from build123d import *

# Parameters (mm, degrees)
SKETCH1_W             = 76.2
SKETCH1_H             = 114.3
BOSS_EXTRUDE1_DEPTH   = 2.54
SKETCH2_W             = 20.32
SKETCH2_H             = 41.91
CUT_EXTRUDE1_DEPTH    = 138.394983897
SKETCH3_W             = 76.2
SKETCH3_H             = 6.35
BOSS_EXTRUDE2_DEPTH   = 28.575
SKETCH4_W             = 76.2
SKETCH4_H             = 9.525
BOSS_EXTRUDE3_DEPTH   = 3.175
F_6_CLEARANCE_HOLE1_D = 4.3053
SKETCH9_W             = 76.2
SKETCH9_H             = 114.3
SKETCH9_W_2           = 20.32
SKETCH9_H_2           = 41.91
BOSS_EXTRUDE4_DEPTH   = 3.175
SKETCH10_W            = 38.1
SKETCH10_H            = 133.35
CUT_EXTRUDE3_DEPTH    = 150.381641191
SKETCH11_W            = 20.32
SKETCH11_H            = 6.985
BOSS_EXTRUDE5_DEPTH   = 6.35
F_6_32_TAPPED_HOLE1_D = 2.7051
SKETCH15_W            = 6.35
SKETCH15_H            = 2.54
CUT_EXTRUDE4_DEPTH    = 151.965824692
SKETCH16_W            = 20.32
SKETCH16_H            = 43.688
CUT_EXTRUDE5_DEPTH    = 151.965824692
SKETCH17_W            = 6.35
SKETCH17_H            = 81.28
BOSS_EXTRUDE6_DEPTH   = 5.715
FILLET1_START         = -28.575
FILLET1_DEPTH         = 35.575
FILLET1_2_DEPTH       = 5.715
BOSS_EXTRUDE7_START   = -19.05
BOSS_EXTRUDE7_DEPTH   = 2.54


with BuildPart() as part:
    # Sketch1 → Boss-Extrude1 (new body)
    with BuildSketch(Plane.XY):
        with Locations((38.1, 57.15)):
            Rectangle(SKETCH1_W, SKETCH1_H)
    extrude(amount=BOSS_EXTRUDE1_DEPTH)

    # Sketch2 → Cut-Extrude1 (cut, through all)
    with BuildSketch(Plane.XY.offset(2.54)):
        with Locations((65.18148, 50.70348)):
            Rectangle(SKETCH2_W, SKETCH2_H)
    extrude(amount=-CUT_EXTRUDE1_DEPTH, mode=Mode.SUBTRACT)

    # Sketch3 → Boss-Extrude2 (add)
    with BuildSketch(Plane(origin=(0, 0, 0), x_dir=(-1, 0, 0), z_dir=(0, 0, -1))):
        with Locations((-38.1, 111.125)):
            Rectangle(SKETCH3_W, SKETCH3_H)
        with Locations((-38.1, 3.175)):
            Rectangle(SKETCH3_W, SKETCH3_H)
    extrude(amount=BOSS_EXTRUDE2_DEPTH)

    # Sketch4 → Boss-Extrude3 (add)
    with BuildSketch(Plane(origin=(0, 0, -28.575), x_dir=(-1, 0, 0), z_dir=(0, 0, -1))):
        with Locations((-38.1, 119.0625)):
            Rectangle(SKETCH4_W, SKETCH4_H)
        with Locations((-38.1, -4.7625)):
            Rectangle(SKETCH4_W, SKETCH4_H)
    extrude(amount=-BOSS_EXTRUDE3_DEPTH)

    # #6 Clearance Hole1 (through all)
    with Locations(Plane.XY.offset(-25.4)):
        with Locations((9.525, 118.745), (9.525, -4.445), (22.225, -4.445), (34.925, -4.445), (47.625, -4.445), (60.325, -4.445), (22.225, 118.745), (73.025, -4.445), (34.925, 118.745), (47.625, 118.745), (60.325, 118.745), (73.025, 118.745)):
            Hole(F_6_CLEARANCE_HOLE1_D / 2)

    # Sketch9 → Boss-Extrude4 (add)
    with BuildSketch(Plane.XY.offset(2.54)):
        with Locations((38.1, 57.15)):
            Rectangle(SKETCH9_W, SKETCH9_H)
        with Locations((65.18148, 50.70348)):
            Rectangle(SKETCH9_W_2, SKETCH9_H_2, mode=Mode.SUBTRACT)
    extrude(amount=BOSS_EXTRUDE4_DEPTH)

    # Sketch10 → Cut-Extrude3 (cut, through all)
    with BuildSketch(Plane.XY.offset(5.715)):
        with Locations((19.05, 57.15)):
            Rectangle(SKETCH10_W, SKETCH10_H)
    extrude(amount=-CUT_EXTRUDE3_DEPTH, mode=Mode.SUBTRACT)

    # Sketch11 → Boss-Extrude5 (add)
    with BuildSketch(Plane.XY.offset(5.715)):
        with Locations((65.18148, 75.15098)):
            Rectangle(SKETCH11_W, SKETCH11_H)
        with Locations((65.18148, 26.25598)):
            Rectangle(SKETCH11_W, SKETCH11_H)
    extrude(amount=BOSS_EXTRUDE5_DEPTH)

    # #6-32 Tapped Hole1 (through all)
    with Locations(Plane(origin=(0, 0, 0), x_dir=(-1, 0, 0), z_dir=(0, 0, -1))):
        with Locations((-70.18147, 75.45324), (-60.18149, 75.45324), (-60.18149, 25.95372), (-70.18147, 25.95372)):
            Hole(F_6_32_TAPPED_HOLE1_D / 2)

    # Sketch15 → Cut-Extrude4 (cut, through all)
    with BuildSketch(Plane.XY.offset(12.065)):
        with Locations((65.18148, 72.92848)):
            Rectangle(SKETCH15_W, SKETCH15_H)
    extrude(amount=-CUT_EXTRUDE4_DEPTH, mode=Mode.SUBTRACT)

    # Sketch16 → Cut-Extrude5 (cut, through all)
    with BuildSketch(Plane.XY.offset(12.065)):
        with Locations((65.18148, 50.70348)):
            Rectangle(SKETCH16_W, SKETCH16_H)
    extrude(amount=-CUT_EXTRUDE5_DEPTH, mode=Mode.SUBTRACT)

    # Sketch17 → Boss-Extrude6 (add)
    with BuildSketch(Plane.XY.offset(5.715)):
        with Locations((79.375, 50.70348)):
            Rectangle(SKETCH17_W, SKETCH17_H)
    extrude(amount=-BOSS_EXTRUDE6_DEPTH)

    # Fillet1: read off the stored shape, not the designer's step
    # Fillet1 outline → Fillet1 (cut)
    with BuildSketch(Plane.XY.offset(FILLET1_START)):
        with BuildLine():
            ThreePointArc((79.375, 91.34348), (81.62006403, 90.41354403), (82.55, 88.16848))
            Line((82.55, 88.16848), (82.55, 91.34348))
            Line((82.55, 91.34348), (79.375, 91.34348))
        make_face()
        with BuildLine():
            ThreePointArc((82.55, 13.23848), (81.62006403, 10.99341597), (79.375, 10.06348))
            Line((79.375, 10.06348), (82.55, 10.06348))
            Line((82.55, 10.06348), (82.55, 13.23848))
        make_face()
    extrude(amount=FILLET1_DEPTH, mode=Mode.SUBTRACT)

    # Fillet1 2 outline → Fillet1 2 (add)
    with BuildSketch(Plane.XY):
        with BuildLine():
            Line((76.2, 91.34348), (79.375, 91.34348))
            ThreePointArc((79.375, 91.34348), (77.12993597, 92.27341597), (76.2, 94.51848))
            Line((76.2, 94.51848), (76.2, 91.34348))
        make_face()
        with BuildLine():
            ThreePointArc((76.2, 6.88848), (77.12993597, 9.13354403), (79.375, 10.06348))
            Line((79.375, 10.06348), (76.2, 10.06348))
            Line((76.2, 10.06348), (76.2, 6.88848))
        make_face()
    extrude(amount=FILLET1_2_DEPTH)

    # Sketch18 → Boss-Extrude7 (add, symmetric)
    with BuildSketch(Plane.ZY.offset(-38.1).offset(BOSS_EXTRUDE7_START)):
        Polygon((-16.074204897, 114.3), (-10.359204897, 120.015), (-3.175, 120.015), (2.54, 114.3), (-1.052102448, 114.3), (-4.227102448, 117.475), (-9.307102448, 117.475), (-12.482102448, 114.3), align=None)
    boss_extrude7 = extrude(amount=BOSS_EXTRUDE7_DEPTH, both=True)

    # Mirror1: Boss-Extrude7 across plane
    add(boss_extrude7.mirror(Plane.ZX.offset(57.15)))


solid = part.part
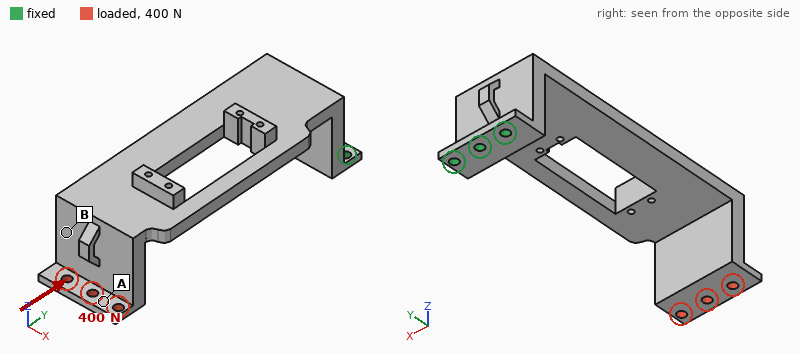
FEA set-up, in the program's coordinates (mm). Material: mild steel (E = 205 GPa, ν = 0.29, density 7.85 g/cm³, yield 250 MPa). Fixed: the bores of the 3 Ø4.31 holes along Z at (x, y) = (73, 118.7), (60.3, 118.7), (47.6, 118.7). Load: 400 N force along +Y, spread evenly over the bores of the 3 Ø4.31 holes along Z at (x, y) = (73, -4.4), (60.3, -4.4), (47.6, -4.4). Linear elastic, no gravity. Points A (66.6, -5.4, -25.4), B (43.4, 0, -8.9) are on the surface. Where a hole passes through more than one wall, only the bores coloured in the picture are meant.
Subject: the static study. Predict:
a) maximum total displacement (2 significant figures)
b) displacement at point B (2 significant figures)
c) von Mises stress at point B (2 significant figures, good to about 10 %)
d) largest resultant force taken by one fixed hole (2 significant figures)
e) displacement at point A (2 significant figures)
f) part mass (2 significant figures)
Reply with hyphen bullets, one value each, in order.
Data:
- 1.1 mm
- 0.84 mm
- 24 MPa
- 150 N
- 0.99 mm
- 320 g
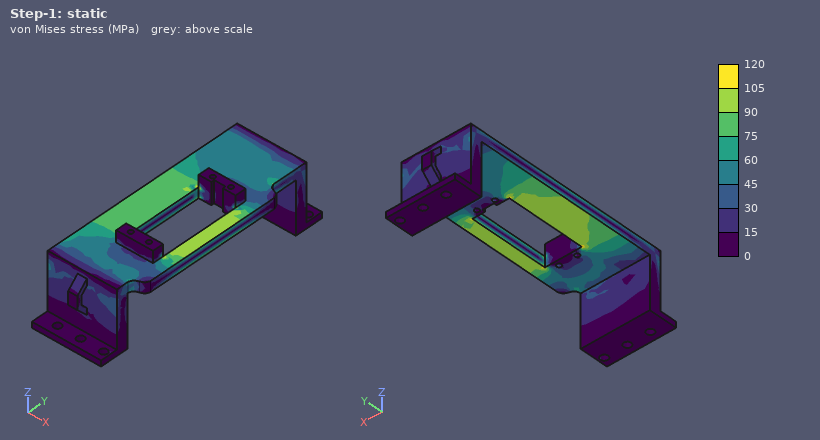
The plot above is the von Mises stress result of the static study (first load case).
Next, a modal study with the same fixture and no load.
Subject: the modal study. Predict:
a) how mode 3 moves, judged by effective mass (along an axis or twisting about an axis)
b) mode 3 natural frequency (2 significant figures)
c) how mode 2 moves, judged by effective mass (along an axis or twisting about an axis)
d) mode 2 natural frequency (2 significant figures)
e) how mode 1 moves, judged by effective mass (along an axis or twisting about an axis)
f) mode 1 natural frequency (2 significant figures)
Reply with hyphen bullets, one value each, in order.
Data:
- along Y
- 680 Hz
- along X
- 370 Hz
- along Z
- 150 Hz
